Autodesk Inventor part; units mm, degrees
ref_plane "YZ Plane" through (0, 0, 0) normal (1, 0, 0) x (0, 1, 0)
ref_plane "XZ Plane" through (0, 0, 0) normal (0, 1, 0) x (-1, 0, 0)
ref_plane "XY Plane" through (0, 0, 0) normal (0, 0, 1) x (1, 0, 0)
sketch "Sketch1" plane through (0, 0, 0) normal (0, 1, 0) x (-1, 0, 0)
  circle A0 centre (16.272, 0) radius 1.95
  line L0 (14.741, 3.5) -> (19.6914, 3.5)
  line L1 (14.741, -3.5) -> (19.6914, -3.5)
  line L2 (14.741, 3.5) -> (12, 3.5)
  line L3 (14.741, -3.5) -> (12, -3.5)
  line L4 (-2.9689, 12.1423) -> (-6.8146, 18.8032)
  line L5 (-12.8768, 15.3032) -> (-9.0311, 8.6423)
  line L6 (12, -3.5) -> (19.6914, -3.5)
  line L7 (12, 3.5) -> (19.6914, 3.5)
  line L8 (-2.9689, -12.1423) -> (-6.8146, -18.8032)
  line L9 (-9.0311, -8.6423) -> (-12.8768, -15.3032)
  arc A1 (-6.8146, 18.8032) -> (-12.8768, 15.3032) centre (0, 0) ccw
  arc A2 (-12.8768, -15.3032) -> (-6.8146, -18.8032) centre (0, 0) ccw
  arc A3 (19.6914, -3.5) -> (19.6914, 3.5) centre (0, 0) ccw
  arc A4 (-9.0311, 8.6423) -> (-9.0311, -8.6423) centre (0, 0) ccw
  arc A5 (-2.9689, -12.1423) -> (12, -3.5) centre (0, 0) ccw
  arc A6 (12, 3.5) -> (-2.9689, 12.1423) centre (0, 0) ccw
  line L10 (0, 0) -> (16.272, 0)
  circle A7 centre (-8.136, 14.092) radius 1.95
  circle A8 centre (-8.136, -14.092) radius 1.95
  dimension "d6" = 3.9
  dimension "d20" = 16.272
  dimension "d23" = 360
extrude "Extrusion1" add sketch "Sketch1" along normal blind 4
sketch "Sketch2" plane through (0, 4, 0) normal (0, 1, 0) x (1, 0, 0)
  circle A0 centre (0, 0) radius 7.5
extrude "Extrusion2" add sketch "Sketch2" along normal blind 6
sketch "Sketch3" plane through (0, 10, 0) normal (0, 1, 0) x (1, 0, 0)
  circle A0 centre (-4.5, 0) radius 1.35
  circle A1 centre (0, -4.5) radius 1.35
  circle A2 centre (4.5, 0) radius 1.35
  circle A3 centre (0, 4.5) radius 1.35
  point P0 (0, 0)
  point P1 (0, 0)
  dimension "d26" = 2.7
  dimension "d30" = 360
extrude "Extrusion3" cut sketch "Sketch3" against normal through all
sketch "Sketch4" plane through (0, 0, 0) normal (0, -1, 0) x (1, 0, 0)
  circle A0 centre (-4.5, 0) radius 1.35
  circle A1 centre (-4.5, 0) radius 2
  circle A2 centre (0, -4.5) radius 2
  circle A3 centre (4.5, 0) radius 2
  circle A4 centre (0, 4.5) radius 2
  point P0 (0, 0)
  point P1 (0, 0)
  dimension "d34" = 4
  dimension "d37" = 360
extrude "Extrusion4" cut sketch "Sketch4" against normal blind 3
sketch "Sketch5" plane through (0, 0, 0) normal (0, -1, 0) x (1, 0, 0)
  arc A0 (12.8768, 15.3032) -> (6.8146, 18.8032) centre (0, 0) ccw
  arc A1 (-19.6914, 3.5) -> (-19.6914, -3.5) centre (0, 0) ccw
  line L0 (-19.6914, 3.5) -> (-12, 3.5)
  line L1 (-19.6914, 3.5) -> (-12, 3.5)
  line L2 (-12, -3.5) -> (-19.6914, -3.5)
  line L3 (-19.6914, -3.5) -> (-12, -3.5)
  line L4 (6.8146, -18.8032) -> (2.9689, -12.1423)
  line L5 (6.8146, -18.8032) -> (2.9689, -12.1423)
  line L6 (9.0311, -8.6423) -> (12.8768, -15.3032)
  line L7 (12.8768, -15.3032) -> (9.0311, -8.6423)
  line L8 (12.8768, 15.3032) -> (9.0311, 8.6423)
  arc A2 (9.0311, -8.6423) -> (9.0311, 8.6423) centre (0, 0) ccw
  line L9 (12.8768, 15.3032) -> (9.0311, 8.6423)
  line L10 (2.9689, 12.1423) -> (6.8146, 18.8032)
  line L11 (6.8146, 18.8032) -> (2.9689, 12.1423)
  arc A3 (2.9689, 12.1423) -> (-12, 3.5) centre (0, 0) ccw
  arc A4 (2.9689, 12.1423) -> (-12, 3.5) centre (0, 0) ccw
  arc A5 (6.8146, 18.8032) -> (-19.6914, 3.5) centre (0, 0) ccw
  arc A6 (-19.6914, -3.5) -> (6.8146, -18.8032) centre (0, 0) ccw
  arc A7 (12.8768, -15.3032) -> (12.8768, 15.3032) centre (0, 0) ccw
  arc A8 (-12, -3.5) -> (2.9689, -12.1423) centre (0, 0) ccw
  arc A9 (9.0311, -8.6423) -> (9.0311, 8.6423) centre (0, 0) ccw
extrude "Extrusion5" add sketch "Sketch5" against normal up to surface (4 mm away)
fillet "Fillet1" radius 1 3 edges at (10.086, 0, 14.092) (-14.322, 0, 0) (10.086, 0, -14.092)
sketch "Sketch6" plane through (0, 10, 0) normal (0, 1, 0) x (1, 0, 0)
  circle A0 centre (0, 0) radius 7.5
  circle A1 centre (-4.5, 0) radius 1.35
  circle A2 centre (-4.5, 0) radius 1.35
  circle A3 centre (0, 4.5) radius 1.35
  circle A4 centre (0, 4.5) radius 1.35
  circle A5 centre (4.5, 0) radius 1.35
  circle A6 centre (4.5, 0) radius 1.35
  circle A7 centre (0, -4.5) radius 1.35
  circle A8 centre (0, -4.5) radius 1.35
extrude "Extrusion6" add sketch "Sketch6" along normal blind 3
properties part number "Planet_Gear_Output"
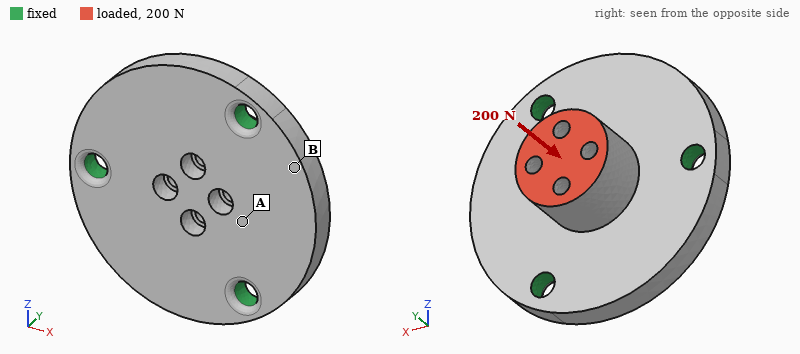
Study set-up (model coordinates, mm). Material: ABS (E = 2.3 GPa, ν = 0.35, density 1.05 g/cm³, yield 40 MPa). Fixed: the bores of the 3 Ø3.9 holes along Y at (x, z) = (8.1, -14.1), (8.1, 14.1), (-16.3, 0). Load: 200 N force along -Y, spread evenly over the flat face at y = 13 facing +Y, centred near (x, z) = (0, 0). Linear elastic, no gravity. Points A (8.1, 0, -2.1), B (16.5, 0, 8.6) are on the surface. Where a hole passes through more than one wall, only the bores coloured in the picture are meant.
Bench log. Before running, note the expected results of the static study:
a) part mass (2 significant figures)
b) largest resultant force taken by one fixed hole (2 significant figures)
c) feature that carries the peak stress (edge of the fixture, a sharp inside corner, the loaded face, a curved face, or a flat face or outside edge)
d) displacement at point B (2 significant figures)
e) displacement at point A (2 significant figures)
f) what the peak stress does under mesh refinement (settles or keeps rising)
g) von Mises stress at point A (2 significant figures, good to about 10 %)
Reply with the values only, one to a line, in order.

6.4 g
67 N
edge of the fixture
13 µm
52 µm
keeps rising
4.1 MPa
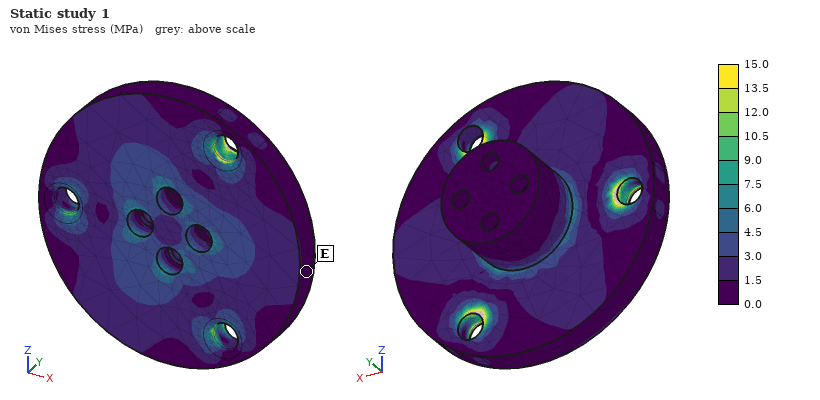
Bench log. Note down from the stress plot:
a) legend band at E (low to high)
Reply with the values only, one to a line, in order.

0.0 to 1.5 MPa
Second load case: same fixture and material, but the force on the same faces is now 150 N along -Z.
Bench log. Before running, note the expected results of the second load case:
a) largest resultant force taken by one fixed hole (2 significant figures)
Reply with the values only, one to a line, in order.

81 N
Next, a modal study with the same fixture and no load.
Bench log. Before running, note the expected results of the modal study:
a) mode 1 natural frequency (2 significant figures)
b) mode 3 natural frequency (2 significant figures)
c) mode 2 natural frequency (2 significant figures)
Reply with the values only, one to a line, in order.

4800 Hz
4900 Hz
4800 Hz
